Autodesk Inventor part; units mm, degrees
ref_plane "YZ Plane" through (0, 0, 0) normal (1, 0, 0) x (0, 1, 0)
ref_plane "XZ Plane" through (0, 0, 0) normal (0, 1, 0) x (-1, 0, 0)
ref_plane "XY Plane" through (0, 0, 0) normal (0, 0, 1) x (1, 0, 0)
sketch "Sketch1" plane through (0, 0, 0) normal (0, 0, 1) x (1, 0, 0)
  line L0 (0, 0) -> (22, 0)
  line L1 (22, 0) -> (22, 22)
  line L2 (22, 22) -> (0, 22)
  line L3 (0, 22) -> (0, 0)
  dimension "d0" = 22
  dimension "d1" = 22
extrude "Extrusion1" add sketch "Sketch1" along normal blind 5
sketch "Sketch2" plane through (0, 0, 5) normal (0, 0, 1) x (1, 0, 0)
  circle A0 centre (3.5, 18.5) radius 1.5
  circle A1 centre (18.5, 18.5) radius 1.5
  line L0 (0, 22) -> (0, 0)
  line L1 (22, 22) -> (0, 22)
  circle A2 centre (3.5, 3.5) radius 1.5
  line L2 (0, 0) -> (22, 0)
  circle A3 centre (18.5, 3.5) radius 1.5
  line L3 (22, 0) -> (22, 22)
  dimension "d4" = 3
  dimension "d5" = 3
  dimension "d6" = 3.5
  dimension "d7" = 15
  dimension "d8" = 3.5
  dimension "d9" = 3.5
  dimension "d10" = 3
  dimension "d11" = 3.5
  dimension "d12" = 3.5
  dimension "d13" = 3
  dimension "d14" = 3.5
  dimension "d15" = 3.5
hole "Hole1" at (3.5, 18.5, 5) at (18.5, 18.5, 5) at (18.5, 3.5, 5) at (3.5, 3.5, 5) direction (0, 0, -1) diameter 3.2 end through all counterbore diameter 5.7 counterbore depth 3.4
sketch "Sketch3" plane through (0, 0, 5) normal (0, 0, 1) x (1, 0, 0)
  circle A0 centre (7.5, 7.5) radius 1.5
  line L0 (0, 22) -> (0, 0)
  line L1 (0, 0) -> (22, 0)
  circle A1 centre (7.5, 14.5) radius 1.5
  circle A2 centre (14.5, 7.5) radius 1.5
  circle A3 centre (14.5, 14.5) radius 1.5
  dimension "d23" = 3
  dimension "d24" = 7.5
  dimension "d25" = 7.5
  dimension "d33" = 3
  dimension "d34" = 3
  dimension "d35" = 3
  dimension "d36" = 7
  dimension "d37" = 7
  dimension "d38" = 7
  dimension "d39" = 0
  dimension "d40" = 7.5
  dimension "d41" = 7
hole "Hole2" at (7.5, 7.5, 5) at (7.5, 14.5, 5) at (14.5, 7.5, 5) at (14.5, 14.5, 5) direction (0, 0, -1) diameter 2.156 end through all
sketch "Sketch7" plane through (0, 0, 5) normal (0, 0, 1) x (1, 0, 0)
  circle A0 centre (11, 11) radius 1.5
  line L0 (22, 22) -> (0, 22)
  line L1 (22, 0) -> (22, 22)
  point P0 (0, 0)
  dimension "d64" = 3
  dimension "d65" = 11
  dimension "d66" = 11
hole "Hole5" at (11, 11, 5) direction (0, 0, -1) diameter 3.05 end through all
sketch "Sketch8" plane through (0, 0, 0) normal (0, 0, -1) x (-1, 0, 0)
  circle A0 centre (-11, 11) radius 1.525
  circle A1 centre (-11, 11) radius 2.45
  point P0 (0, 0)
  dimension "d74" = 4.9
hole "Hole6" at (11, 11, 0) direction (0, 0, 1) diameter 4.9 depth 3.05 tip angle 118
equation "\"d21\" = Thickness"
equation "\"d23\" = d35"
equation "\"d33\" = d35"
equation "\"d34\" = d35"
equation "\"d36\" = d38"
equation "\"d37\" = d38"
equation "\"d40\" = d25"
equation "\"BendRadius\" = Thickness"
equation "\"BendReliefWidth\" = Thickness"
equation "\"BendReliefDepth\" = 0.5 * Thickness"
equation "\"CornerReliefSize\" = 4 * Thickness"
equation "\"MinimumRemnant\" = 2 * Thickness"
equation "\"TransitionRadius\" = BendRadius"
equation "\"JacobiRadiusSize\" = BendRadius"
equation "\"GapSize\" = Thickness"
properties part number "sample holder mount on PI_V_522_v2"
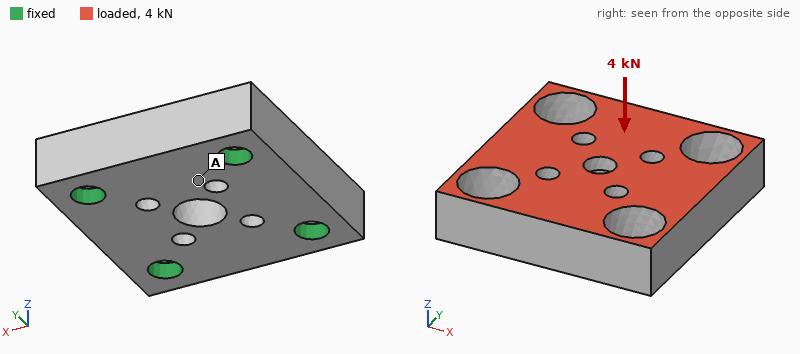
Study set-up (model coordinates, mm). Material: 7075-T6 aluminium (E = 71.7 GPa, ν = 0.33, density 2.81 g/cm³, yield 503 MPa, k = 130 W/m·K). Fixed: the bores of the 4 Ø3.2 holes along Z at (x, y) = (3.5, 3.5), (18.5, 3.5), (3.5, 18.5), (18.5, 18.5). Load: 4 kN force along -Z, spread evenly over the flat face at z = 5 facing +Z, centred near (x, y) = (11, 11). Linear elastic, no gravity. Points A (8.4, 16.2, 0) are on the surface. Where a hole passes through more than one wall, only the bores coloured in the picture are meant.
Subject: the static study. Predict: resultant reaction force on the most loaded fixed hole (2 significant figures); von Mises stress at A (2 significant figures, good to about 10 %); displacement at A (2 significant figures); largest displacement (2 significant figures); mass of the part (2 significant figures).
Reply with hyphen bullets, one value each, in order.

- 1.1 kN
- 27 MPa
- 10.0 µm
- 13 µm
- 5.3 g
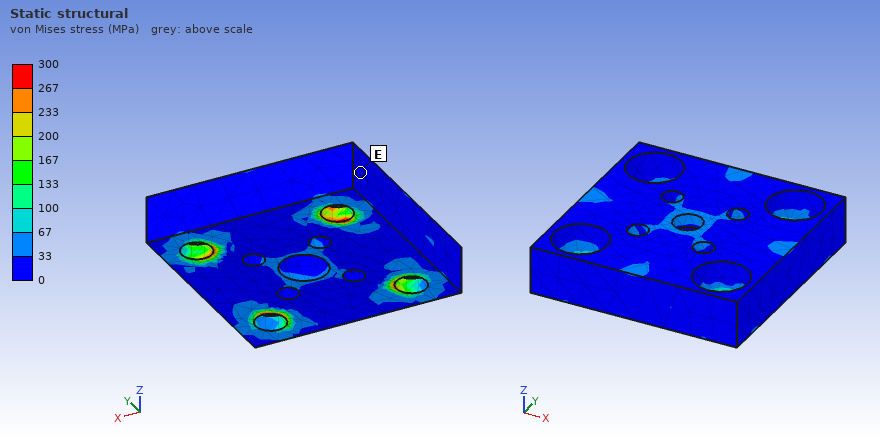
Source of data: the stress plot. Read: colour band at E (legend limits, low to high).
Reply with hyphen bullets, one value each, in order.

- 0 to 33 MPa
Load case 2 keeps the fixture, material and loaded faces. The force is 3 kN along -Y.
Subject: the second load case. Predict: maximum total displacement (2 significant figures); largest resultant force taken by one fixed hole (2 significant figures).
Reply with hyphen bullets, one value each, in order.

- 11 µm
- 860 N
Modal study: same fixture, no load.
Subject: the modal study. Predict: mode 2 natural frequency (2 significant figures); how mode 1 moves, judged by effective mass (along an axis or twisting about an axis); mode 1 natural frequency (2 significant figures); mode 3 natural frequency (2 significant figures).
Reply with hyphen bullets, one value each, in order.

- 56 kHz
- along Z
- 46 kHz
- 56 kHz
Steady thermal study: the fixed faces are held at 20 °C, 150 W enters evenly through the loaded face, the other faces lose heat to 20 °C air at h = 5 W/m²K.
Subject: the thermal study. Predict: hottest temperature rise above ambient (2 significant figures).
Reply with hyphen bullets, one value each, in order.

- 54 K
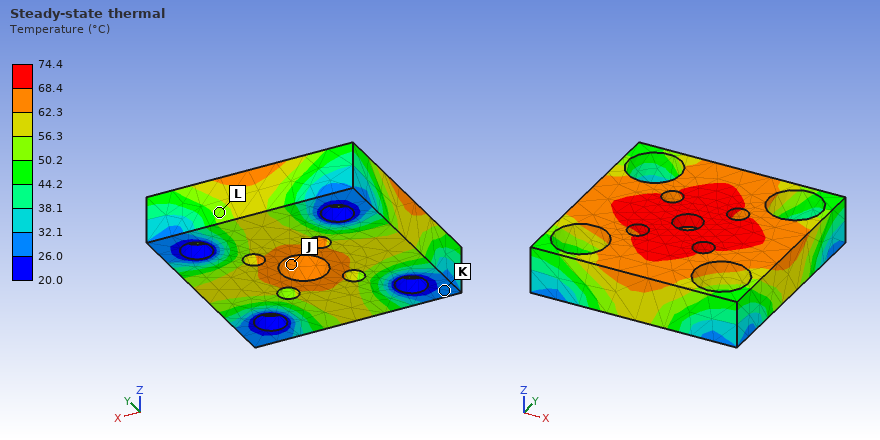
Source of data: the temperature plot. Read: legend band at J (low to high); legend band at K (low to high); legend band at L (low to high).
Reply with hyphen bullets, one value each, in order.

- 62.3 to 68.4 °C
- 26.0 to 32.1 °C
- 50.2 to 56.3 °C
